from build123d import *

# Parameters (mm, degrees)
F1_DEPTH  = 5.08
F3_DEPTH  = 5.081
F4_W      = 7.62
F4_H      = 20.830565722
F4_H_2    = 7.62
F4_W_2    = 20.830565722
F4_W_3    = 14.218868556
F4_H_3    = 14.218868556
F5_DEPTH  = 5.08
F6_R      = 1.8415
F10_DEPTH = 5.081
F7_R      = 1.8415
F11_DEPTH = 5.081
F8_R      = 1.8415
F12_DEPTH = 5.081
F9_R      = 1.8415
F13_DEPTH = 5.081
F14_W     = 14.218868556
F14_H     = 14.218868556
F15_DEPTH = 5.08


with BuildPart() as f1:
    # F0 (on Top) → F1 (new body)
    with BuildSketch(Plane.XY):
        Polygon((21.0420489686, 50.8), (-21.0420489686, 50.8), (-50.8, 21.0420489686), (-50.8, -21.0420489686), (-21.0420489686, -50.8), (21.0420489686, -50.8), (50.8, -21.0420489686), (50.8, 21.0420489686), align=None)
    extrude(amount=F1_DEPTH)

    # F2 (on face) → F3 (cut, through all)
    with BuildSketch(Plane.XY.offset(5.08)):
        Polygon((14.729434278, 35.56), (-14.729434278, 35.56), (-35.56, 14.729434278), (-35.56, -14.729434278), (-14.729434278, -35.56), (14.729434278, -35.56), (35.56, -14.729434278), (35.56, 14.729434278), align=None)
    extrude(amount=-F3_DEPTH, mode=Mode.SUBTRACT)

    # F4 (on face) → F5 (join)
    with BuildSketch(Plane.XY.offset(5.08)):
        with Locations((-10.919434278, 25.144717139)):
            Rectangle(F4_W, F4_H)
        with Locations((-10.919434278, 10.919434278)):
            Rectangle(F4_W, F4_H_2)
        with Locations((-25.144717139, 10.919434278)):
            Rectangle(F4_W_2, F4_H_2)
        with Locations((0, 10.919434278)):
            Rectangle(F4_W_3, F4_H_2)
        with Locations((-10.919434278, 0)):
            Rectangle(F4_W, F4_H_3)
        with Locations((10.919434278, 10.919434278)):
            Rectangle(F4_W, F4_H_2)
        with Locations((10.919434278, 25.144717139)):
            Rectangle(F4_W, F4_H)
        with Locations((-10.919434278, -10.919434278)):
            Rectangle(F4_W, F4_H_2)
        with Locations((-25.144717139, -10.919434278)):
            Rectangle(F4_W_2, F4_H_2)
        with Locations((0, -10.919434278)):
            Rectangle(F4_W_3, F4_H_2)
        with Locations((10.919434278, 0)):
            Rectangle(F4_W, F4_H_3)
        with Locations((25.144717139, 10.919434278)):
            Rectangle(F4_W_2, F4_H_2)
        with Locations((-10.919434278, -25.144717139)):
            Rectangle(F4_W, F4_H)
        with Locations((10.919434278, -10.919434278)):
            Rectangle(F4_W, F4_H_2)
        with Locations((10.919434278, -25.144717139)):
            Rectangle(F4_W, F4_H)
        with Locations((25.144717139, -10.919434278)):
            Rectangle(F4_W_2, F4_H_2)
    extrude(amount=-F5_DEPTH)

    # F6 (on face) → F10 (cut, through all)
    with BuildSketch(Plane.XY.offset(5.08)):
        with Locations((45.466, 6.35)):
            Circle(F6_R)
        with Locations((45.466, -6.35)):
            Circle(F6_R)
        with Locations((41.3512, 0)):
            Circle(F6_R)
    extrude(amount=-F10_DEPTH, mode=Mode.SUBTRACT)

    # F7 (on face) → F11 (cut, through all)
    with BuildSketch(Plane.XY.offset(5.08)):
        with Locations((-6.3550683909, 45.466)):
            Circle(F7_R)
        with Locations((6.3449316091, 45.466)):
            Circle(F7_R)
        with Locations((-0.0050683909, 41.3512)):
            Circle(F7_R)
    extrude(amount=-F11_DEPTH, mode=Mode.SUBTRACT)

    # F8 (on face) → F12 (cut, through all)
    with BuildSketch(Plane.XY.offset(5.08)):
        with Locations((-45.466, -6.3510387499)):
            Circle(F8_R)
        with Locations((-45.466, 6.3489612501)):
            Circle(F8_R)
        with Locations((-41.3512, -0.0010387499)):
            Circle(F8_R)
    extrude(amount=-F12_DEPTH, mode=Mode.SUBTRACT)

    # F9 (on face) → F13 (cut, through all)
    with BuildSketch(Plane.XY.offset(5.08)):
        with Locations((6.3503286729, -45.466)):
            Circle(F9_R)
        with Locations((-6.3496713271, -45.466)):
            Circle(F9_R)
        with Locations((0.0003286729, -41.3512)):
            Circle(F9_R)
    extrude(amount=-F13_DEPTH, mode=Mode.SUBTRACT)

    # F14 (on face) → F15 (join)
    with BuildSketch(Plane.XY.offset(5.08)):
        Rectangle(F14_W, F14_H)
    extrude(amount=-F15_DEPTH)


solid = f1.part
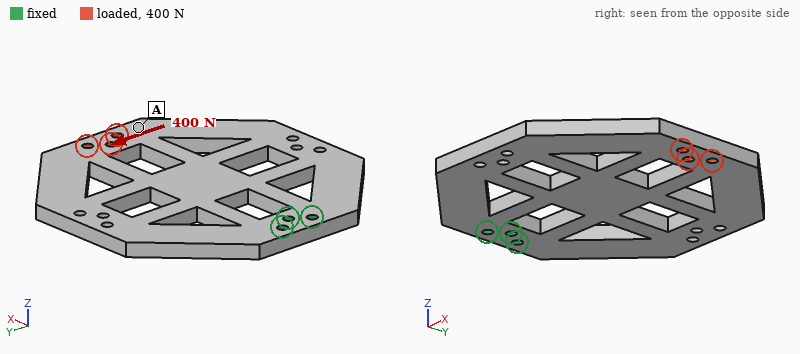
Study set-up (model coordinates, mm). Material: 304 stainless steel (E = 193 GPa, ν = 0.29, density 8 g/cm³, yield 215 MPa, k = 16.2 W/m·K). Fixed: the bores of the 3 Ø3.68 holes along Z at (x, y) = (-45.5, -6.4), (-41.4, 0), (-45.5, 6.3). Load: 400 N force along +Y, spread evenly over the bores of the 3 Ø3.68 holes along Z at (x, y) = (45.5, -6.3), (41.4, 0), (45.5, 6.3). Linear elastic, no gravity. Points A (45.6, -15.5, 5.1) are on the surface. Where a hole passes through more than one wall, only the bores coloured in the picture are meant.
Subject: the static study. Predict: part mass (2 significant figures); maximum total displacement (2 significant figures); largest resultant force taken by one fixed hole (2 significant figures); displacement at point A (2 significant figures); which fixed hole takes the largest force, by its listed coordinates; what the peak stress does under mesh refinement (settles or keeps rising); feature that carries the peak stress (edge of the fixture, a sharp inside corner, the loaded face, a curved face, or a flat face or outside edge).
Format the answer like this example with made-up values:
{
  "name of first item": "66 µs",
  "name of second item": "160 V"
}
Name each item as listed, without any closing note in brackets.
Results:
{
  "part mass": "260 g",
  "maximum total displacement": "55 µm",
  "largest resultant force taken by one fixed hole": "1.9 kN",
  "displacement at point A": "52 µm",
  "which fixed hole takes the largest force, by its listed coordinates": "(-41.4, 0)",
  "what the peak stress does under mesh refinement": "keeps rising",
  "feature that carries the peak stress": "edge of the fixture"
}
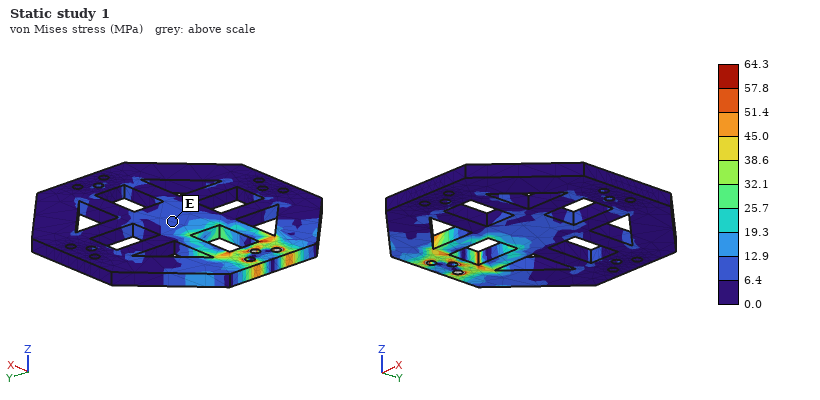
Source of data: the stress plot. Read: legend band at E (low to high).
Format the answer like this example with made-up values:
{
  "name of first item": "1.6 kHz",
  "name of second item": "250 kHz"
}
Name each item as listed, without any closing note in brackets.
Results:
{
  "legend band at E": "6.4 to 12.9 MPa"
}
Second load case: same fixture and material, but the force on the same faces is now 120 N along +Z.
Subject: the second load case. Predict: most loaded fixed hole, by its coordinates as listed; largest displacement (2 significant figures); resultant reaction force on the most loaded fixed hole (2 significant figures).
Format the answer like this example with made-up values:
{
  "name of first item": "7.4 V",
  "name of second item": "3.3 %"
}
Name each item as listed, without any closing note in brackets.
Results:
{
  "most loaded fixed hole, by its coordinates as listed": "(-41.4, 0)",
  "largest displacement": "0.39 mm",
  "resultant reaction force on the most loaded fixed hole": "400 N"
}
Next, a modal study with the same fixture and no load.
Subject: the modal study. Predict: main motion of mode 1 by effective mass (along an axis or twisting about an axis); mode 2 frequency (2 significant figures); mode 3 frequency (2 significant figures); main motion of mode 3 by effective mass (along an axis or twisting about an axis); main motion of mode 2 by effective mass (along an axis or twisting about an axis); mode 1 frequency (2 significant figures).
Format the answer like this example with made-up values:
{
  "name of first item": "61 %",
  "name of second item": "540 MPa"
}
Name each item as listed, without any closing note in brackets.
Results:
{
  "main motion of mode 1 by effective mass": "along Z",
  "mode 2 frequency": "710 Hz",
  "mode 3 frequency": "1300 Hz",
  "main motion of mode 3 by effective mass": "along Y",
  "main motion of mode 2 by effective mass": "twisting about X",
  "mode 1 frequency": "350 Hz"
}
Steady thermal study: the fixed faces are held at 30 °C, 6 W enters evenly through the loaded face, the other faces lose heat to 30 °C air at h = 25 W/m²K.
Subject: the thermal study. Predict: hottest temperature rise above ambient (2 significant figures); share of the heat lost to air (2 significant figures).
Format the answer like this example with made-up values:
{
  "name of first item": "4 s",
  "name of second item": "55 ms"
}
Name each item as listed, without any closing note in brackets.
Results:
{
  "hottest temperature rise above ambient": "62 K",
  "share of the heat lost to air": "94 %"
}
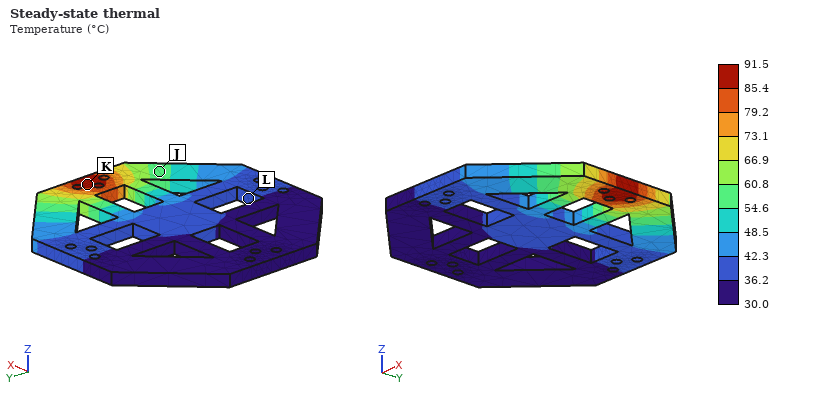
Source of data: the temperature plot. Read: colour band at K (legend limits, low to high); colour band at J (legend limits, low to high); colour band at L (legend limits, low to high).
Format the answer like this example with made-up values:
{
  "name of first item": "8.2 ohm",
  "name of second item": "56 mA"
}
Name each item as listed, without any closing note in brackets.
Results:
{
  "colour band at K": "85.4 to 91.5 °C",
  "colour band at J": "54.6 to 60.8 °C",
  "colour band at L": "36.2 to 42.3 °C"
}
